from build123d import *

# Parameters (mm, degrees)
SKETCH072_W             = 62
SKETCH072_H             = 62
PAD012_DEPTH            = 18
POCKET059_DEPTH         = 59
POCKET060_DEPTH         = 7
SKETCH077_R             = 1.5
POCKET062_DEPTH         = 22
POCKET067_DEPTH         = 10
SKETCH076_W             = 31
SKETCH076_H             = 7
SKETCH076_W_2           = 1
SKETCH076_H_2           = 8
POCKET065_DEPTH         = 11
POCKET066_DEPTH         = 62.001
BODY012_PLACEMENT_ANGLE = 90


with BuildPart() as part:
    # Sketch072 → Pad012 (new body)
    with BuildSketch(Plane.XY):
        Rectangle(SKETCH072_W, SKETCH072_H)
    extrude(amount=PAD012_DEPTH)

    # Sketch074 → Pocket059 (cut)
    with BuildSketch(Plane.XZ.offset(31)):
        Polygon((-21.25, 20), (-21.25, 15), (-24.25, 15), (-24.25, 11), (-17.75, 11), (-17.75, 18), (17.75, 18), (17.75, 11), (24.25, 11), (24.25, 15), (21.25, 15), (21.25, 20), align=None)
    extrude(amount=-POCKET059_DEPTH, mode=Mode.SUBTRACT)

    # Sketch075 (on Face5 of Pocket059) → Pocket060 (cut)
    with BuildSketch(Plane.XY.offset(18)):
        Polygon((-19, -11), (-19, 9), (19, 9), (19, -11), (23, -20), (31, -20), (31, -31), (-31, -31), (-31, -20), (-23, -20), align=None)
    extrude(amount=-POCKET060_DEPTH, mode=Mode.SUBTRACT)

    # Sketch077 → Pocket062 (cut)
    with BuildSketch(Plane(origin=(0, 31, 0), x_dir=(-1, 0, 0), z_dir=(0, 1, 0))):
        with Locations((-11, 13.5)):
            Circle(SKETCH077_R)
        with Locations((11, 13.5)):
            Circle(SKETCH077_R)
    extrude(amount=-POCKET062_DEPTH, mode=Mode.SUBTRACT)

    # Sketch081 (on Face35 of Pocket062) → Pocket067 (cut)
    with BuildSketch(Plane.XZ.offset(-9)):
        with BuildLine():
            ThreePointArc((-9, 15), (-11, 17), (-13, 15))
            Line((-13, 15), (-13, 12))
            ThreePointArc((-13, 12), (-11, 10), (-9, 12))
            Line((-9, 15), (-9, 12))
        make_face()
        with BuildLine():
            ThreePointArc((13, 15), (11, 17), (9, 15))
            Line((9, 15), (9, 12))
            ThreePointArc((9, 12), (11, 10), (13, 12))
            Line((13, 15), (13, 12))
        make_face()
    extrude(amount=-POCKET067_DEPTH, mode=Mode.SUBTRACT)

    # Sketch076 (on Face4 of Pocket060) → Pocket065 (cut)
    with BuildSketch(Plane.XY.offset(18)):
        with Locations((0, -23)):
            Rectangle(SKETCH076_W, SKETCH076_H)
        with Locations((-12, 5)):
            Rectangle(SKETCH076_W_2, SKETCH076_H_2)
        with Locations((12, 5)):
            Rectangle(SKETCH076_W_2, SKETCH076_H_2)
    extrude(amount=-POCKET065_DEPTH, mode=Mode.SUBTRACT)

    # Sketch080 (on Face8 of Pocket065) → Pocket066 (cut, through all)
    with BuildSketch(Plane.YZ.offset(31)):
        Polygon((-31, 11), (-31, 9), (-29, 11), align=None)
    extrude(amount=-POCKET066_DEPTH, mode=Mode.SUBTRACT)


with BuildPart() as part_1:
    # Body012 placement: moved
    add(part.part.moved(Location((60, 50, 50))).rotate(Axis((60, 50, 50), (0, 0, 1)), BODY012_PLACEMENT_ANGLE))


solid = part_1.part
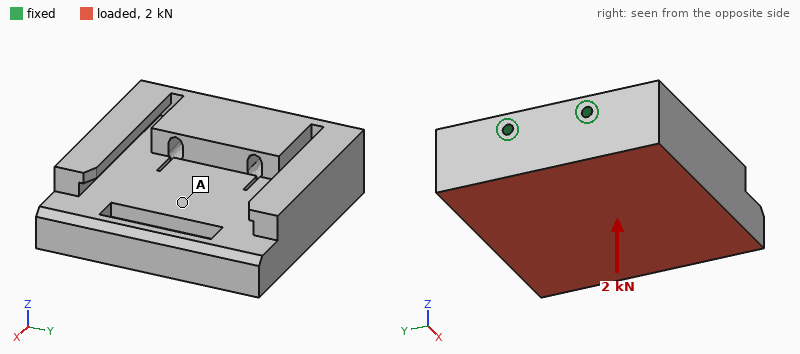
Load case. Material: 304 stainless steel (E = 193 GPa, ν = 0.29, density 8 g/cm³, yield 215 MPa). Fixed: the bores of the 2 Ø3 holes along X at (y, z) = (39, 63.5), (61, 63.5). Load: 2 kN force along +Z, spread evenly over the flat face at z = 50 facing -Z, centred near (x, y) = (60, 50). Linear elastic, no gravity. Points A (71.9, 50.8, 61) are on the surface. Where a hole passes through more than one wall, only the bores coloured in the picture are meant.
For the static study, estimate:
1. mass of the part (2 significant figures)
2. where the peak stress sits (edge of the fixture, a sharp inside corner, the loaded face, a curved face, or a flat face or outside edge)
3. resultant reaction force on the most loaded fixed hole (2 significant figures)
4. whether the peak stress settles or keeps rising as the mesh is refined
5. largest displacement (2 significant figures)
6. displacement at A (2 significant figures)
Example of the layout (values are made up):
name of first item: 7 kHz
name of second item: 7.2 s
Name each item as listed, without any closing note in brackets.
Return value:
mass of the part: 420 g
where the peak stress sits: edge of the fixture
resultant reaction force on the most loaded fixed hole: 1.0 kN
whether the peak stress settles or keeps rising as the mesh is refined: keeps rising
largest displacement: 34 µm
displacement at A: 20 µm
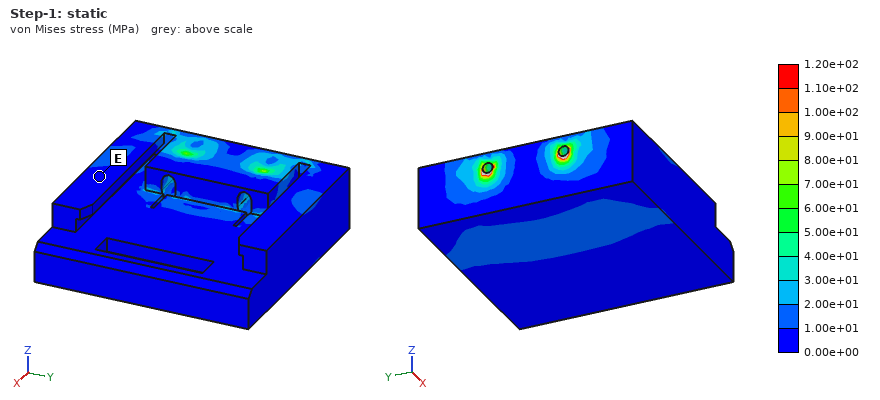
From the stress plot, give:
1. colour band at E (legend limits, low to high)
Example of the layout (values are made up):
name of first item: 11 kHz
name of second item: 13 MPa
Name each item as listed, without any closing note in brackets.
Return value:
colour band at E: 0.00e+00 to 1.00e+01 MPa
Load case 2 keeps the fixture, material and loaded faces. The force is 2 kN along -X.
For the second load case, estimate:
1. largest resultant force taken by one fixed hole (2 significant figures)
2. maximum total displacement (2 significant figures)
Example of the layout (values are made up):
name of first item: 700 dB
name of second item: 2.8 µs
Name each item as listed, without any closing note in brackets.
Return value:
largest resultant force taken by one fixed hole: 1.0 kN
maximum total displacement: 16 µm
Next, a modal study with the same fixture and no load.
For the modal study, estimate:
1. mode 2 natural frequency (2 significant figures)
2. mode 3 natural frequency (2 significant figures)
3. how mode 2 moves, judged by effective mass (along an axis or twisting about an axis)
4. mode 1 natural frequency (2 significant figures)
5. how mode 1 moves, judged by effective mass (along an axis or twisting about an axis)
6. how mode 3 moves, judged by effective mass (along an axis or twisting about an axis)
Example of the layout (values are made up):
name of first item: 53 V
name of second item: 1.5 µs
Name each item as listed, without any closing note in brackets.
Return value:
mode 2 natural frequency: 4400 Hz
mode 3 natural frequency: 5200 Hz
how mode 2 moves, judged by effective mass: along Y
mode 1 natural frequency: 2500 Hz
how mode 1 moves, judged by effective mass: along Z
how mode 3 moves, judged by effective mass: along Y
